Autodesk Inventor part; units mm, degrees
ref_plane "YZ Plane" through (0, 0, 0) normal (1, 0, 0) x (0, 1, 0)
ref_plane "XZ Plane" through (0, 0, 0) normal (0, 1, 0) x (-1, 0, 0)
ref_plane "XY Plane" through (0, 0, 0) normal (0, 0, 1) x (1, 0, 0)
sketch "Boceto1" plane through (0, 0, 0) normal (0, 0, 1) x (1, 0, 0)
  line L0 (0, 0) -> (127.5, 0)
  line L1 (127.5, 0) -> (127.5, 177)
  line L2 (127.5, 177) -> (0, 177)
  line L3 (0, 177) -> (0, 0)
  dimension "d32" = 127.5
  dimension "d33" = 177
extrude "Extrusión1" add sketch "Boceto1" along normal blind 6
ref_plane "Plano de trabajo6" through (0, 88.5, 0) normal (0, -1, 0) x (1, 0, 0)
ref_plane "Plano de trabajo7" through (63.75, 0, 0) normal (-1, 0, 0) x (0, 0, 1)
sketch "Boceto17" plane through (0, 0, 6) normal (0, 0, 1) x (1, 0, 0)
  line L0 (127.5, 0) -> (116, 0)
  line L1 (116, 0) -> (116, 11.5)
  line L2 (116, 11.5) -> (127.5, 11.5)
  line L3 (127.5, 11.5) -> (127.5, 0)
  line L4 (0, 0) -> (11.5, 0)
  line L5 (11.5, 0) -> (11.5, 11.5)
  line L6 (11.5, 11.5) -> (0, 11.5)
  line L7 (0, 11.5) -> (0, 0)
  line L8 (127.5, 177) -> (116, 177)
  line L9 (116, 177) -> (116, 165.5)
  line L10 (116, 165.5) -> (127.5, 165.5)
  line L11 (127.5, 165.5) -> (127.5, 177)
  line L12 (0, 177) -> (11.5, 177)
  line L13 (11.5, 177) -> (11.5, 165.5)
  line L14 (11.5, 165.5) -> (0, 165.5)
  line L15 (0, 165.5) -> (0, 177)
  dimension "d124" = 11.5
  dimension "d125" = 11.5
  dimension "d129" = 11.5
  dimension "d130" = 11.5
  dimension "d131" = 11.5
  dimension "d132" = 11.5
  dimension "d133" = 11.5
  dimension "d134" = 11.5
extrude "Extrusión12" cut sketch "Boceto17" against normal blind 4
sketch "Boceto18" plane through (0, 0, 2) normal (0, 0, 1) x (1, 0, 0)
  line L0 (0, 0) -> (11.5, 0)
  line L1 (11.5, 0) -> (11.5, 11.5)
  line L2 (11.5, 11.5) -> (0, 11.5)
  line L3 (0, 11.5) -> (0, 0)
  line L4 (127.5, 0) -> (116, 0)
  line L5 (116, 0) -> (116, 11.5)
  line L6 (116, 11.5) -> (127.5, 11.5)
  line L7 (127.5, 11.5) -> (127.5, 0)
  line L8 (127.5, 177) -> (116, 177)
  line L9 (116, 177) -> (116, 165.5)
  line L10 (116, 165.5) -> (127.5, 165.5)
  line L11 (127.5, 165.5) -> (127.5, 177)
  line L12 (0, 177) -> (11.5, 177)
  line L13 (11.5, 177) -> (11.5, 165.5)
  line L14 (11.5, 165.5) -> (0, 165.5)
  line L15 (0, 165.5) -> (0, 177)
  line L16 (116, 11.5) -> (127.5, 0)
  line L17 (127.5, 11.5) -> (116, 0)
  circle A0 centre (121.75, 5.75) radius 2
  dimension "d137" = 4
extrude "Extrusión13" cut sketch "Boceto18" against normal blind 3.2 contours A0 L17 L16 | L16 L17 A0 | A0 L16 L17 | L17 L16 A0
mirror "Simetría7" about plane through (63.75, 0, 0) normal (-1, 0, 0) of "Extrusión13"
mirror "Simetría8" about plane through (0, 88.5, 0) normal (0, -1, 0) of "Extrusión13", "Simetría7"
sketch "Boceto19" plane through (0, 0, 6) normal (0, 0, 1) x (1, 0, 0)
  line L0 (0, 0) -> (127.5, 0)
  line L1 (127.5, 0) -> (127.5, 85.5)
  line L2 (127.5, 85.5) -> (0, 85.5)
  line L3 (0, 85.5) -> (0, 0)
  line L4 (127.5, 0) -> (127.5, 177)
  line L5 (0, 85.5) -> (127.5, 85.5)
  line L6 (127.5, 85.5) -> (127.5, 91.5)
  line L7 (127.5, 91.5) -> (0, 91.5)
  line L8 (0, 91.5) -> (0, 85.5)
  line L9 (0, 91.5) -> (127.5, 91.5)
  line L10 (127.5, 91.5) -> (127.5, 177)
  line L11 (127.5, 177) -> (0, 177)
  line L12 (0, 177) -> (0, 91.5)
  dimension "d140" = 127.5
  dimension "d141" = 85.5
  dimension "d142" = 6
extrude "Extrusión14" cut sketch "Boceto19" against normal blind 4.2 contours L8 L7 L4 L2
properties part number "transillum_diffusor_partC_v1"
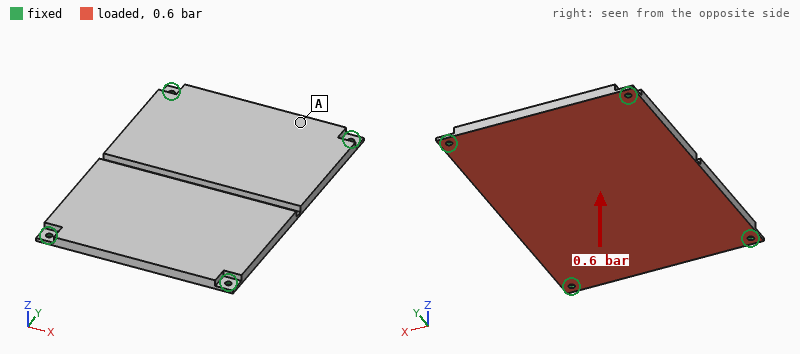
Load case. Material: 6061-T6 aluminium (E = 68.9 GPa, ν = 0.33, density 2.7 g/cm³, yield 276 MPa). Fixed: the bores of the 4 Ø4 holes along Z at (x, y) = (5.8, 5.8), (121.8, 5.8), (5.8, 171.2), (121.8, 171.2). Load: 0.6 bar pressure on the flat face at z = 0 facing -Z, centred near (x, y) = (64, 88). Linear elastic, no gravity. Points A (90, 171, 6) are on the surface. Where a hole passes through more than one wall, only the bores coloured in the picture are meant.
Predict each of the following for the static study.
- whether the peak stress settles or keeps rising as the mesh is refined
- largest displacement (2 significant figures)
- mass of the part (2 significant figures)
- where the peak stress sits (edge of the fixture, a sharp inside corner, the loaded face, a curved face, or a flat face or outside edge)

keeps rising
0.90 mm
350 g
edge of the fixture
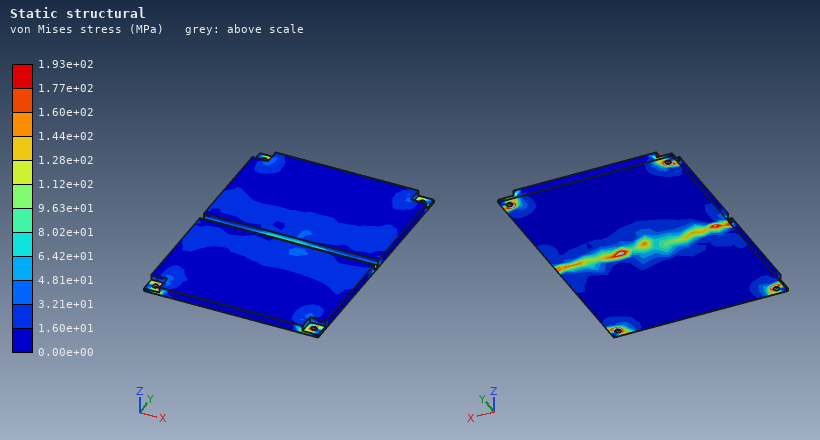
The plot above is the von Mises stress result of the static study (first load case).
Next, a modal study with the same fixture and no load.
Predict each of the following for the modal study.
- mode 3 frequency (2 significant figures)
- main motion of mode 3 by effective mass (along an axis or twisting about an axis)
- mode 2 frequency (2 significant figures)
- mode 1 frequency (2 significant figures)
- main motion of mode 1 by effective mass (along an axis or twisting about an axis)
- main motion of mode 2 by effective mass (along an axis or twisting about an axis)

1500 Hz
twisting about X
1100 Hz
400 Hz
along Z
twisting about Y
